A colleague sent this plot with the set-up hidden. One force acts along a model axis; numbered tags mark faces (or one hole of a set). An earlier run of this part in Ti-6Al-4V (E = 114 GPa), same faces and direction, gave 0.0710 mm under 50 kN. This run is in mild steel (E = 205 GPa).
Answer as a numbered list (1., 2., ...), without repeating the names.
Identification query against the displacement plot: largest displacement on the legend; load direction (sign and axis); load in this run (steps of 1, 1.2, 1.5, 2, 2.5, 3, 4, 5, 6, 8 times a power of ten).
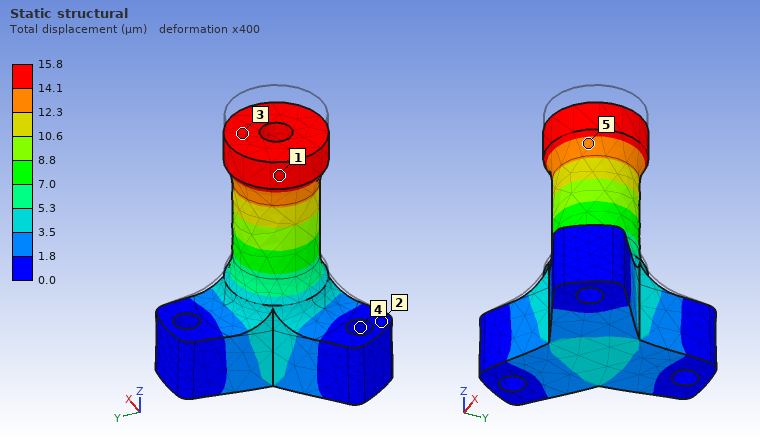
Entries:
1. 15.8 µm
2. -Z
3. 20 kN
